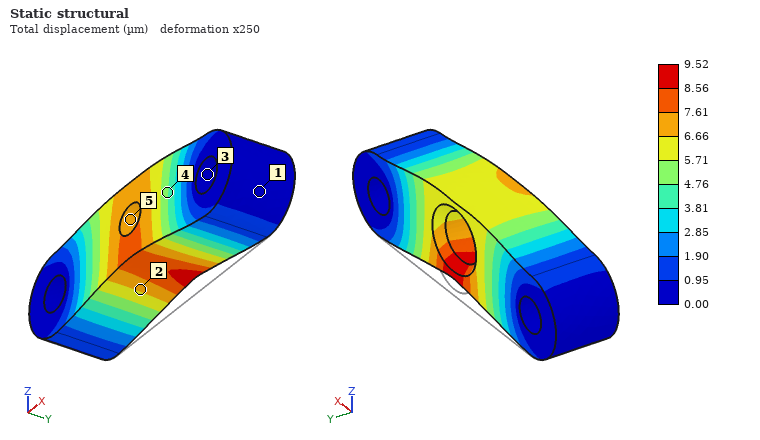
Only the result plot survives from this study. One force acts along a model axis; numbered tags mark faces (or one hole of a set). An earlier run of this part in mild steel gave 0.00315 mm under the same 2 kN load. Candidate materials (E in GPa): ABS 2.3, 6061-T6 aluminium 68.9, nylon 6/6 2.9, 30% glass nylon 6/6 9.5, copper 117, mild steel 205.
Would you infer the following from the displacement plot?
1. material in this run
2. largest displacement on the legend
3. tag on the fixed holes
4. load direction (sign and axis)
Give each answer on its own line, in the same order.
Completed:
6061-T6 aluminium
9.52 µm
3
+Z
